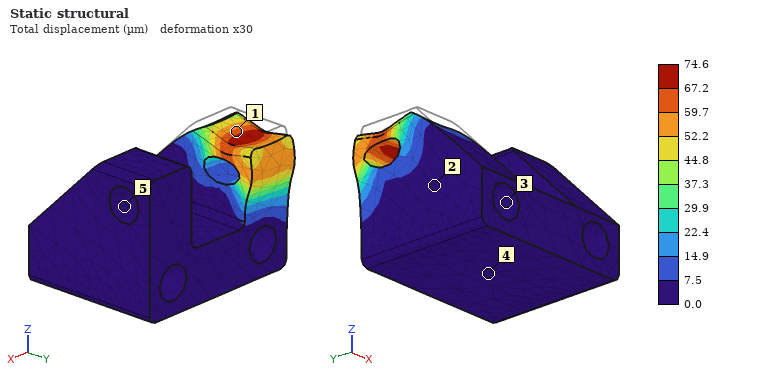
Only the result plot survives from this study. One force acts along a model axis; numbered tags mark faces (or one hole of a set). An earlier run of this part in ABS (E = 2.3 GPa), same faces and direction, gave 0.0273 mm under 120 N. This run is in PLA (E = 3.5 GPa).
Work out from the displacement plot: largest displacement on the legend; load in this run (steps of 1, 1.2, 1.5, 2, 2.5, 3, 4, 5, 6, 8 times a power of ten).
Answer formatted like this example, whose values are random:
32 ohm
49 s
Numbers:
74.6 µm
500 N
